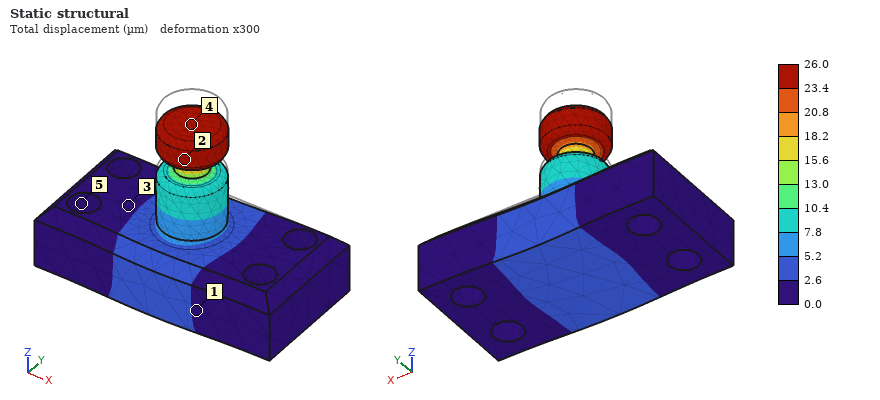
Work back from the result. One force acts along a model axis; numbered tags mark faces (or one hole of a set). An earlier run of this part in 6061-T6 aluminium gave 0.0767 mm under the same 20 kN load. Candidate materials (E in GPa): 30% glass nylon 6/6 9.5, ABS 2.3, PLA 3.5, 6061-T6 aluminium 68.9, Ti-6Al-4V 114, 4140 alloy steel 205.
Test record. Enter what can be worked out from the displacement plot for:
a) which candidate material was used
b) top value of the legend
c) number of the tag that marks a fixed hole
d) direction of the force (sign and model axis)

4140 alloy steel
26.0 µm
5
-Z
